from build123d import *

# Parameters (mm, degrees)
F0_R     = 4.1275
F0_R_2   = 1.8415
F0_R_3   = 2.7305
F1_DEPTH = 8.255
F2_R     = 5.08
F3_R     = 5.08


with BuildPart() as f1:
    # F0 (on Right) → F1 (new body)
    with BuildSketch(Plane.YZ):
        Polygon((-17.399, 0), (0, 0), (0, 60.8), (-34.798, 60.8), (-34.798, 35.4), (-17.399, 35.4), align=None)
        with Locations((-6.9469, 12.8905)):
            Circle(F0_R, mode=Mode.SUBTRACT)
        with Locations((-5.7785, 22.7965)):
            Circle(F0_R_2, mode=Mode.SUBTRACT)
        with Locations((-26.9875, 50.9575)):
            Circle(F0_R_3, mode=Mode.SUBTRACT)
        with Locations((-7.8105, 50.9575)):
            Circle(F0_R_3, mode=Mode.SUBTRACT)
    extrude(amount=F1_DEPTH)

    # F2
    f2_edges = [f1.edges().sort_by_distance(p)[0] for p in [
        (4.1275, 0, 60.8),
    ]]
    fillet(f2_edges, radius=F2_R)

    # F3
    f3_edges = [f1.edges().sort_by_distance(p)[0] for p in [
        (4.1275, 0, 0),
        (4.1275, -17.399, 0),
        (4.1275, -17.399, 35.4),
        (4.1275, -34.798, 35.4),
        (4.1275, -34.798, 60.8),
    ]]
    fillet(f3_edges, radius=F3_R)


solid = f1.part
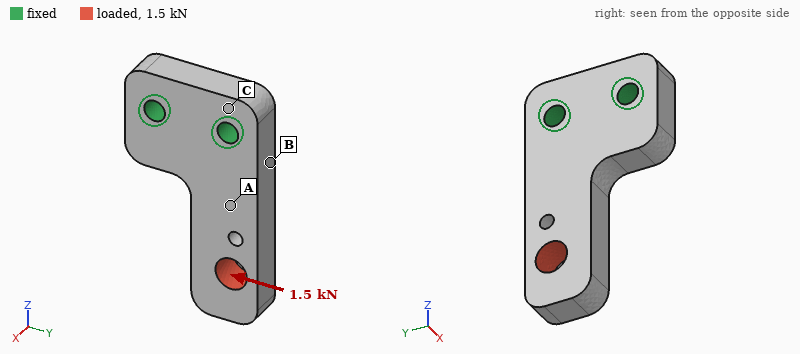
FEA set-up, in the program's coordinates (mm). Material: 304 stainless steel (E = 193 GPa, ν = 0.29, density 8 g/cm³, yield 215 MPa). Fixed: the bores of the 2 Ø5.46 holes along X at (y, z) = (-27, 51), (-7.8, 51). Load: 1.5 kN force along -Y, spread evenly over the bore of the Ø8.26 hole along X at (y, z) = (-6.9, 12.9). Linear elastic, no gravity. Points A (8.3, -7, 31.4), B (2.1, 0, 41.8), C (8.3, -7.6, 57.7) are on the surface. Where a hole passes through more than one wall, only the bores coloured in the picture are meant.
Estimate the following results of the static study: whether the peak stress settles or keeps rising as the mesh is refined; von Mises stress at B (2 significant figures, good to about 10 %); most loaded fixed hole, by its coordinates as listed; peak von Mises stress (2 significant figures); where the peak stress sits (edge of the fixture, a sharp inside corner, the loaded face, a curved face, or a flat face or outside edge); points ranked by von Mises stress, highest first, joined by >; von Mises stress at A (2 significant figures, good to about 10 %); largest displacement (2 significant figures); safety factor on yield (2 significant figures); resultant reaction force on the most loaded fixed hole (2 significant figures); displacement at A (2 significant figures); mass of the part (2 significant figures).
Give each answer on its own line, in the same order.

settles
53 MPa
(-27, 51)
130 MPa
a curved face
B > A > C
27 MPa
39 µm
1.7
2.8 kN
6.1 µm
90 g
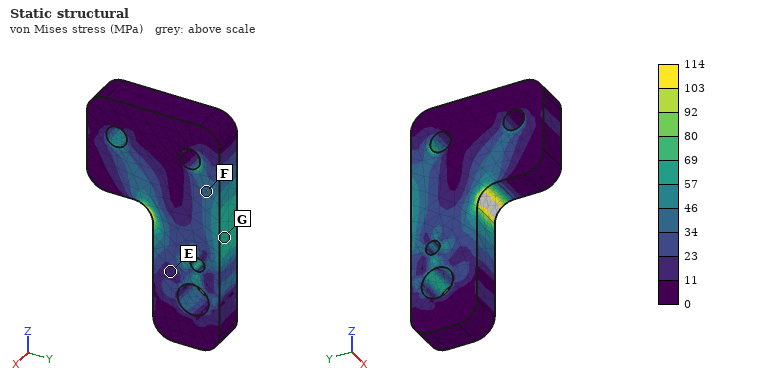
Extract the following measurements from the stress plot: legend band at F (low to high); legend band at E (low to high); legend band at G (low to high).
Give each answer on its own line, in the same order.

34 to 46 MPa
11 to 23 MPa
57 to 69 MPa
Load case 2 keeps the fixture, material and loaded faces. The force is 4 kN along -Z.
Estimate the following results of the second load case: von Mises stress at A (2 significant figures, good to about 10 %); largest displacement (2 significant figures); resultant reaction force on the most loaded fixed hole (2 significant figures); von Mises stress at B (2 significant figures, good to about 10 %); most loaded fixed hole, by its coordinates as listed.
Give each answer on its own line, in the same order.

28 MPa
17 µm
3.9 kN
38 MPa
(-7.8, 51)
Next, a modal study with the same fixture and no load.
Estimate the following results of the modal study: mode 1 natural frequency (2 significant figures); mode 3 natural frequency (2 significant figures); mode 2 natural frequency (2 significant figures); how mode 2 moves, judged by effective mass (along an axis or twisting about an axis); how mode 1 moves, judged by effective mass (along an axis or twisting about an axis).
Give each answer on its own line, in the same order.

3100 Hz
13 kHz
7100 Hz
along Y
along X
